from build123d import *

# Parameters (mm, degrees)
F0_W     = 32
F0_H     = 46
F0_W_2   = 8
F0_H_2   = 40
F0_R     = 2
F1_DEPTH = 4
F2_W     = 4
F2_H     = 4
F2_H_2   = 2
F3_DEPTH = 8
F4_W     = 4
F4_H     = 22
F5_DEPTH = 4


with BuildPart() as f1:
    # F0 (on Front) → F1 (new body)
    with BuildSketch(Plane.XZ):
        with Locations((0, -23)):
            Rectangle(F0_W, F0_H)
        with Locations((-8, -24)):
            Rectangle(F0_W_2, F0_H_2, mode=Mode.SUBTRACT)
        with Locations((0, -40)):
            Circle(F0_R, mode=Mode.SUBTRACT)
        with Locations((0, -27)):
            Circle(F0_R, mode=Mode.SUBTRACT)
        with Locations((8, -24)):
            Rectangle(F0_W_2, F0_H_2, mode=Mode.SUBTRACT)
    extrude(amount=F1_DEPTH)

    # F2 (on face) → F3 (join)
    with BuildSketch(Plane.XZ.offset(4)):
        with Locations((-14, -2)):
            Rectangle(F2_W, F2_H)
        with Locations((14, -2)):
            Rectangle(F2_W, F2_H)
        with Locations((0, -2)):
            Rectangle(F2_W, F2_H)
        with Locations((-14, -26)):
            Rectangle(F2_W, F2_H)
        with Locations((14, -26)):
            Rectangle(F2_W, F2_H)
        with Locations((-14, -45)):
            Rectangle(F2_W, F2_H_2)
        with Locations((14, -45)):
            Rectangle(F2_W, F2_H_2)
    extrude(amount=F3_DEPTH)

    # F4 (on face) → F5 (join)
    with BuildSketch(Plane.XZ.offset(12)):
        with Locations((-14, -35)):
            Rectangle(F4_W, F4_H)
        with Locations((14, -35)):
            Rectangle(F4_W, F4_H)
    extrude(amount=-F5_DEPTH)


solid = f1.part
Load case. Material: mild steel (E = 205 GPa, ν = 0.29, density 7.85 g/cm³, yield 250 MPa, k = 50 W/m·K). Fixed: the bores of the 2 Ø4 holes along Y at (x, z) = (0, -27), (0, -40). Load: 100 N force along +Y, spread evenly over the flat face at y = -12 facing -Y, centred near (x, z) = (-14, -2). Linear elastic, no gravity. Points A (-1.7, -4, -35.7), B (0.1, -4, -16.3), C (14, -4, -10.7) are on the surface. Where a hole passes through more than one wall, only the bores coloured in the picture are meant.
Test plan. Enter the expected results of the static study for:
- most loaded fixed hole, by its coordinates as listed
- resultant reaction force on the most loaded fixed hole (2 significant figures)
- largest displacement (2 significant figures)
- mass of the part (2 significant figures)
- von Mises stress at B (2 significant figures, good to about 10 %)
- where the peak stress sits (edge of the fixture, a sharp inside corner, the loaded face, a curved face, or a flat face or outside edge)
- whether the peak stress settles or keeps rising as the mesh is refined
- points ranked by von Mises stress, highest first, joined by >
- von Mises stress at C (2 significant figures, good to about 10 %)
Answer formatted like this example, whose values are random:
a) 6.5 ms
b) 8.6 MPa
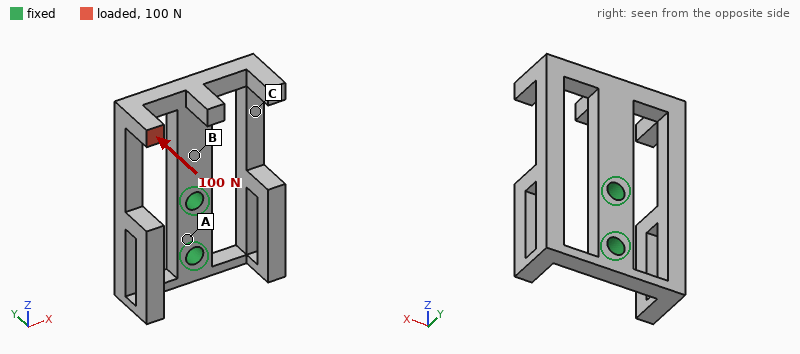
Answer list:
a) (0, -27)
b) 110 N
c) 0.11 mm
d) 35 g
e) 75 MPa
f) edge of the fixture
g) keeps rising
h) B > C > A
i) 25 MPa
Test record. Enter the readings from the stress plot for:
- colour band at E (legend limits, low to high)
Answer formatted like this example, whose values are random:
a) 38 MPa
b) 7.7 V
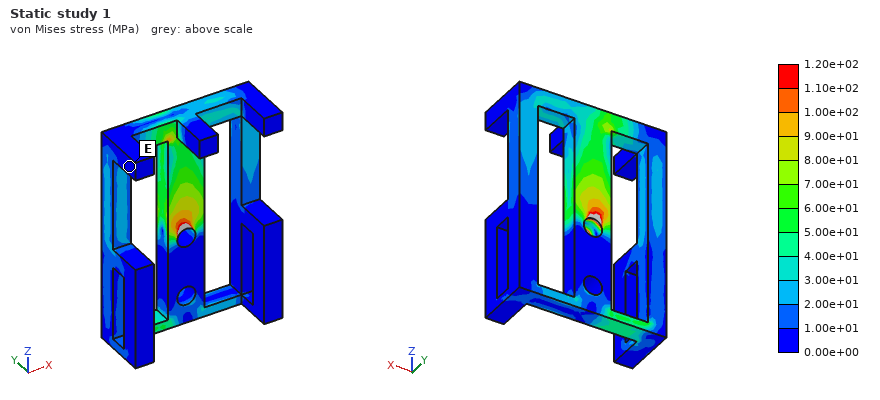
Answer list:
a) 0.00e+00 to 1.00e+01 MPa
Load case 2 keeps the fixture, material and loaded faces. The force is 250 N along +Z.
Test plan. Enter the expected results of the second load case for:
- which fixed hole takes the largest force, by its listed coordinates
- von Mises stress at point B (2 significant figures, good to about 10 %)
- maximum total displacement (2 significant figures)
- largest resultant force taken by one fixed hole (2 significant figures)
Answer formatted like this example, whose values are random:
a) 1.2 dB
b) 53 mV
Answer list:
a) (0, -27)
b) 63 MPa
c) 0.13 mm
d) 200 N
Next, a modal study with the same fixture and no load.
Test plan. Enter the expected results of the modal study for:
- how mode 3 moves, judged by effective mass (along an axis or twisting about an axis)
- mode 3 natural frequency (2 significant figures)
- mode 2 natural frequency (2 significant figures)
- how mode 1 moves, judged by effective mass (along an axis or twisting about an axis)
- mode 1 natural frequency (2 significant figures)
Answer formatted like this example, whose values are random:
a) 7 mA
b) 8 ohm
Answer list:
a) along X
b) 3200 Hz
c) 2300 Hz
d) along Y
e) 2200 Hz
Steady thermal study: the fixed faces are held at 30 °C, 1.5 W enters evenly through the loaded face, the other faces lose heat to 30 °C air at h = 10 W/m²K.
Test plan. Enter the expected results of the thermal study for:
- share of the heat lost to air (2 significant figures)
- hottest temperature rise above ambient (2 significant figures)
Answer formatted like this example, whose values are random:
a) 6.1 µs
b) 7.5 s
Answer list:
a) 24 %
b) 41 K
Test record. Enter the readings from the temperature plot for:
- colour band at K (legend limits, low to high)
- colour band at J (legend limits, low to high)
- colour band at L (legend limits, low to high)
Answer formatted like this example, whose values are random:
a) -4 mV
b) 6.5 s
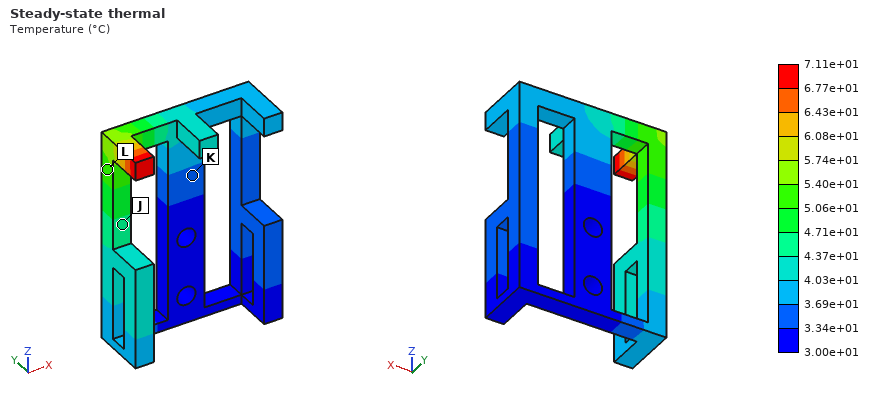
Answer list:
a) 3.34e+01 to 3.69e+01 °C
b) 4.37e+01 to 4.71e+01 °C
c) 5.06e+01 to 5.40e+01 °C
